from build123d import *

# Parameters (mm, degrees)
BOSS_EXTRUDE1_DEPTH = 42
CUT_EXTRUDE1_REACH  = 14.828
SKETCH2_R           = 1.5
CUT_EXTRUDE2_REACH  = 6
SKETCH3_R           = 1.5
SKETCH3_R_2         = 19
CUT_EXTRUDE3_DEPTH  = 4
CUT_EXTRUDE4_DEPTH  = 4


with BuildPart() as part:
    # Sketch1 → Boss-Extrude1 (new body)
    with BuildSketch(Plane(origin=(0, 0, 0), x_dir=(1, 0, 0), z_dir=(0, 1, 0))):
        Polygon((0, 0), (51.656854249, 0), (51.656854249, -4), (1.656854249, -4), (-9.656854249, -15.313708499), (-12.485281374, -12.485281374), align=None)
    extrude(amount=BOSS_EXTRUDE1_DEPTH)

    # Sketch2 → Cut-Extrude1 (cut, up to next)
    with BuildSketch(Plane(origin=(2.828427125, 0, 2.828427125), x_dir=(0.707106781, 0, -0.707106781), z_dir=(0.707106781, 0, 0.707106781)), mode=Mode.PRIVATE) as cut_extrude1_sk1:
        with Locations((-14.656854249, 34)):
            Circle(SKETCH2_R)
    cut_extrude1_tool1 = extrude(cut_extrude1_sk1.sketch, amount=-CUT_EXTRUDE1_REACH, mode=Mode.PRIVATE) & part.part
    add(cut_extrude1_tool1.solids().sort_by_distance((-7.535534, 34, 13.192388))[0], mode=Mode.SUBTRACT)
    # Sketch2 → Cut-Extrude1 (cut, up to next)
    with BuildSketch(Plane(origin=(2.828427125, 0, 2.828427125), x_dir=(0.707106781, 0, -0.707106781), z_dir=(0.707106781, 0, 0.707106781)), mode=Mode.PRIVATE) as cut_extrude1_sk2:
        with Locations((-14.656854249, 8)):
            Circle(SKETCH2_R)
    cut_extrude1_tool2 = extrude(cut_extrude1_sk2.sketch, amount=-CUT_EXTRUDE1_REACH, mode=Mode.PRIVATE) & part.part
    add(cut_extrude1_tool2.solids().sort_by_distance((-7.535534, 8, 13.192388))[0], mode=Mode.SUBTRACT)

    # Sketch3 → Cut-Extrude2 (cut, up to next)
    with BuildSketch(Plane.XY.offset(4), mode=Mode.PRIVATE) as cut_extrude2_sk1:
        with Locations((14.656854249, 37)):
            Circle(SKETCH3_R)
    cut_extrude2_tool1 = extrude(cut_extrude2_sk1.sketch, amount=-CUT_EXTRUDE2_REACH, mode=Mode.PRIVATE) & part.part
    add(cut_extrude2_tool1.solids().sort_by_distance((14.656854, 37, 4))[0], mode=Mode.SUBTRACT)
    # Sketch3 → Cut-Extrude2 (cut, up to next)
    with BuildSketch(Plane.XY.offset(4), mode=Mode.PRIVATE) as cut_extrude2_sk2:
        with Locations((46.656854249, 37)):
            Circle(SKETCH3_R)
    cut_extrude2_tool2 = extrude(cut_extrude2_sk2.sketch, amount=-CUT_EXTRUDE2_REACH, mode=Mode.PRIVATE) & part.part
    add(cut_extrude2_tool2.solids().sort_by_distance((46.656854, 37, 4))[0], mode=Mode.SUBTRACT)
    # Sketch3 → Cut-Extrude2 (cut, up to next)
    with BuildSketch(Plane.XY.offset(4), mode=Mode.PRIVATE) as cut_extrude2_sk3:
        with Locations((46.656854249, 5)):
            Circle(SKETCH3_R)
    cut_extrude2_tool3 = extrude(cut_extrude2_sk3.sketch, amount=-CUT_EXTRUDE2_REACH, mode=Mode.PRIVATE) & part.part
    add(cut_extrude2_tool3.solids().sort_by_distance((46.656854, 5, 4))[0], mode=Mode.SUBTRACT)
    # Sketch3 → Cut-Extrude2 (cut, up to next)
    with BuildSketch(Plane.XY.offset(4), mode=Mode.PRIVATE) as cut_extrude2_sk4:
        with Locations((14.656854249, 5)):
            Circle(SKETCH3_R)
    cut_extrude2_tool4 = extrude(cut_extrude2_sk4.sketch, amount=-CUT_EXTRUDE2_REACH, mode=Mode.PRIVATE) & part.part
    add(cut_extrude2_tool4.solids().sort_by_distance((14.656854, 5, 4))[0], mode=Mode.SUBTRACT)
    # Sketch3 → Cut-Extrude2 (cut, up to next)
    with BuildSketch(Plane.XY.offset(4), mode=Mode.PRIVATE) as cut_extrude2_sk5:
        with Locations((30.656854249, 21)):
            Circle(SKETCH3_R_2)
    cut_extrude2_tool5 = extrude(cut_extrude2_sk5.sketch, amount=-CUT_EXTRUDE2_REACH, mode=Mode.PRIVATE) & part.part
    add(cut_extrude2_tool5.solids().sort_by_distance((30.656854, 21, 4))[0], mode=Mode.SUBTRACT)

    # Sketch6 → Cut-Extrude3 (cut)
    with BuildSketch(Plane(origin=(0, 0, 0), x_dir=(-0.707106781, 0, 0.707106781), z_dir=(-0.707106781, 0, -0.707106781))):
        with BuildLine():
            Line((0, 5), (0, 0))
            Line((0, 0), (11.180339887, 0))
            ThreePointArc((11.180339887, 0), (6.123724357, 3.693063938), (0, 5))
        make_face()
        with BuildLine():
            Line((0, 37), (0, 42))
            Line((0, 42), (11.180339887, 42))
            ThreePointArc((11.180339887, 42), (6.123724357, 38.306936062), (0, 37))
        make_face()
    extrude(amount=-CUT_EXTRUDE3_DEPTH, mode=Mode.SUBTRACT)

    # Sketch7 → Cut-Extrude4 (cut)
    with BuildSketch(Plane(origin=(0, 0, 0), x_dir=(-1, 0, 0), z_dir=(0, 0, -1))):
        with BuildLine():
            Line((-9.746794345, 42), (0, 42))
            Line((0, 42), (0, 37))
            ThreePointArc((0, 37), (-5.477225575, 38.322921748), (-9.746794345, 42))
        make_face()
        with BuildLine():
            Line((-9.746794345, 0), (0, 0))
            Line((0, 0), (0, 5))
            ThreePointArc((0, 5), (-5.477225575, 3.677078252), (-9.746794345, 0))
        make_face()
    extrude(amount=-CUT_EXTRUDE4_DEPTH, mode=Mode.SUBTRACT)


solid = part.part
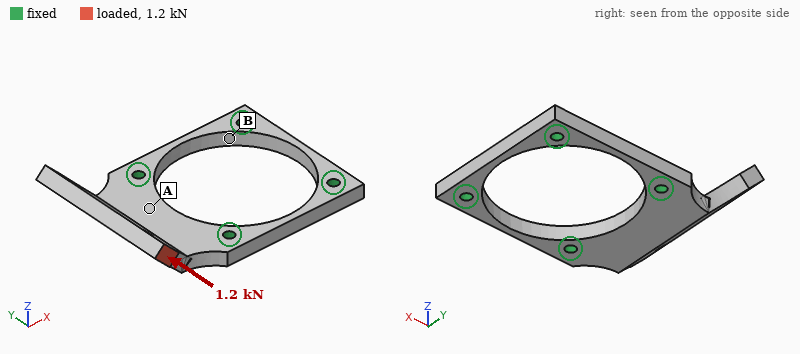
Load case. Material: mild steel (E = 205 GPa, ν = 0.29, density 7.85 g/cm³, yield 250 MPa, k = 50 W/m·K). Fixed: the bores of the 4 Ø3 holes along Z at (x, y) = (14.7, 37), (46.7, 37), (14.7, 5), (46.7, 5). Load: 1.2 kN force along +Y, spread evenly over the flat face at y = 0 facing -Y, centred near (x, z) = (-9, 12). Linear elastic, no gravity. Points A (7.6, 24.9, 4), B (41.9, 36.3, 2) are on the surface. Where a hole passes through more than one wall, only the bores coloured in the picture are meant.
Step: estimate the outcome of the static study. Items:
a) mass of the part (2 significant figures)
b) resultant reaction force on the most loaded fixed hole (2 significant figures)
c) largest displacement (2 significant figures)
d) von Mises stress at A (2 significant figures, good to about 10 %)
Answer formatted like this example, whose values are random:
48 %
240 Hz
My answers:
48 g
1.1 kN
38 µm
55 MPa
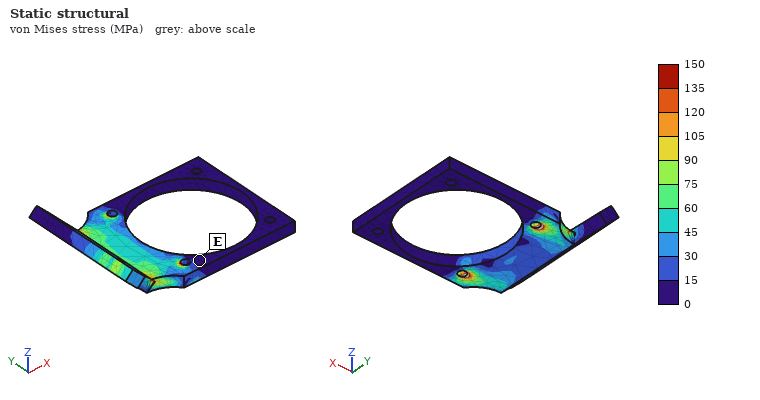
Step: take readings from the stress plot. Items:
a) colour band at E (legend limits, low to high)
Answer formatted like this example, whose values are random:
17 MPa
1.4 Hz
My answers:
0 to 15 MPa
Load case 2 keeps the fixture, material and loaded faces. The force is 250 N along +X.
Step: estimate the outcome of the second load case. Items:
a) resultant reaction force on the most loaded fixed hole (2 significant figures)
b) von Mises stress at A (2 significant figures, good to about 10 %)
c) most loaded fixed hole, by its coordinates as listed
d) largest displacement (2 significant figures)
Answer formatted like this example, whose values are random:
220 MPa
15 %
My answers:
300 N
19 MPa
(14.7, 5)
58 µm
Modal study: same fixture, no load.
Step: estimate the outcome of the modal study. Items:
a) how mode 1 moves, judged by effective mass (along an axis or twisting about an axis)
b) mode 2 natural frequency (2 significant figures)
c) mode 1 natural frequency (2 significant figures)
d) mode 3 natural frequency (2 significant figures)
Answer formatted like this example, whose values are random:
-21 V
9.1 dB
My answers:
along Z
6600 Hz
2900 Hz
13 kHz
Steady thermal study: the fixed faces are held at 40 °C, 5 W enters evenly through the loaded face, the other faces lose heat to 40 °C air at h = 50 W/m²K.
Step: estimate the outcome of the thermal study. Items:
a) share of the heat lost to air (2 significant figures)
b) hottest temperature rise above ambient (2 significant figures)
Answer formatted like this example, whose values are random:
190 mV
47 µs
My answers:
33 %
52 K
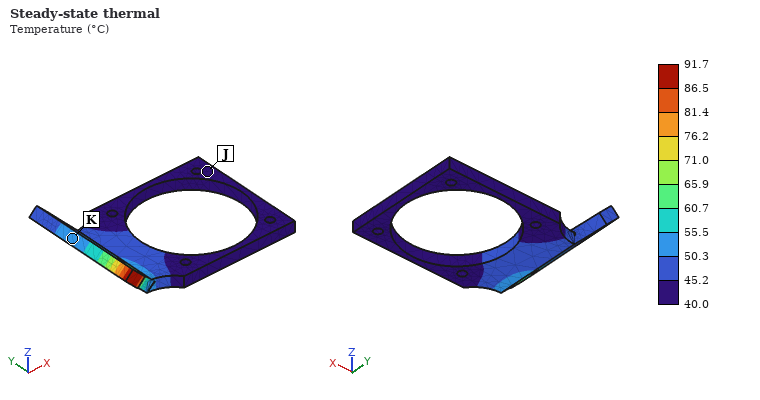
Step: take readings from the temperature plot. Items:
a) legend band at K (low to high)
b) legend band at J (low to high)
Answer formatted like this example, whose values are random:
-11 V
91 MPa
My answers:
50.3 to 55.5 °C
40.0 to 45.2 °C
